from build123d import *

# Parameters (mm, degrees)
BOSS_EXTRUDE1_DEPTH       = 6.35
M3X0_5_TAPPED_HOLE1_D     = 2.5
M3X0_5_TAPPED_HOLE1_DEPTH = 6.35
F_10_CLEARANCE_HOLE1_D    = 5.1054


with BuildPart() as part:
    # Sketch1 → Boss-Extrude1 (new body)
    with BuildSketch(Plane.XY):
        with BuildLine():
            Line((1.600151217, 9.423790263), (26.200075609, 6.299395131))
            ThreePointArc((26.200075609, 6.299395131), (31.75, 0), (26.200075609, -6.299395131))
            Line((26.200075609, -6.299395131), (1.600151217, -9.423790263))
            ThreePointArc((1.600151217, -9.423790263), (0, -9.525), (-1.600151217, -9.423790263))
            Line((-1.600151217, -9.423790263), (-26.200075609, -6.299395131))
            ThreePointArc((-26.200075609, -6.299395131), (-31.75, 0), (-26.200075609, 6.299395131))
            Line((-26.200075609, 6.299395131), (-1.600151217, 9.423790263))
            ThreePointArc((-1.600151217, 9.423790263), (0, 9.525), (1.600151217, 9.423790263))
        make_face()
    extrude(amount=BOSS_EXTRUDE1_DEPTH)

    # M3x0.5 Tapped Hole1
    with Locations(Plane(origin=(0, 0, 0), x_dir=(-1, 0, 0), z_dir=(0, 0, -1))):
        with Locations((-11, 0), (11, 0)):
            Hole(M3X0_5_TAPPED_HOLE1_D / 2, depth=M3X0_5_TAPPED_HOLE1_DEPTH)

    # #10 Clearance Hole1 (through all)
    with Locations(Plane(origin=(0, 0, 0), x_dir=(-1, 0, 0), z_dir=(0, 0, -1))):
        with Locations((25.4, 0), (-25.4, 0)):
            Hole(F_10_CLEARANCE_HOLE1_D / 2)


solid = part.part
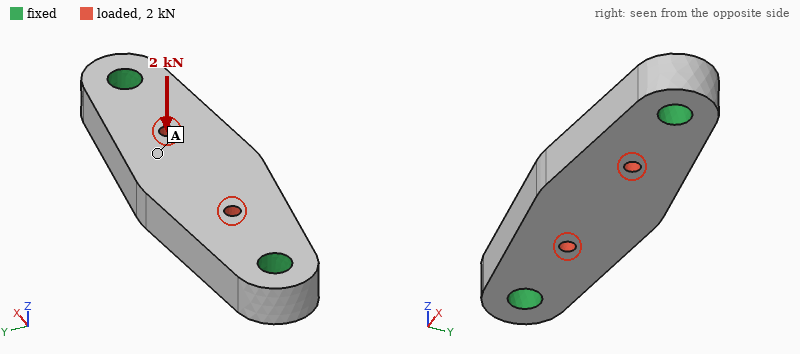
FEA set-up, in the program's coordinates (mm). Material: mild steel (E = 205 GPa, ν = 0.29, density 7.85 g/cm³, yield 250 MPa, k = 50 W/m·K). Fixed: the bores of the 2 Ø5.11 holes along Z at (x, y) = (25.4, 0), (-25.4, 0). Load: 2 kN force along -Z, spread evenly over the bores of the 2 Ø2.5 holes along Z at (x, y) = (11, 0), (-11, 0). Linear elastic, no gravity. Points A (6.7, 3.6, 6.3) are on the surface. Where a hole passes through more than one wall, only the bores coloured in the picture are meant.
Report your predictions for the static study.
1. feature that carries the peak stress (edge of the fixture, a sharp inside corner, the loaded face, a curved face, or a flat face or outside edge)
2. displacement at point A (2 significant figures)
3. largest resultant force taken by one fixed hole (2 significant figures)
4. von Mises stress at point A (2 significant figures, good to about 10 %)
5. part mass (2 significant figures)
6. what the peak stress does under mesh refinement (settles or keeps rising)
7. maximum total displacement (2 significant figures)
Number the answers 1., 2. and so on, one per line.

1. edge of the fixture
2. 11 µm
3. 1.0 kN
4. 35 MPa
5. 44 g
6. keeps rising
7. 12 µm
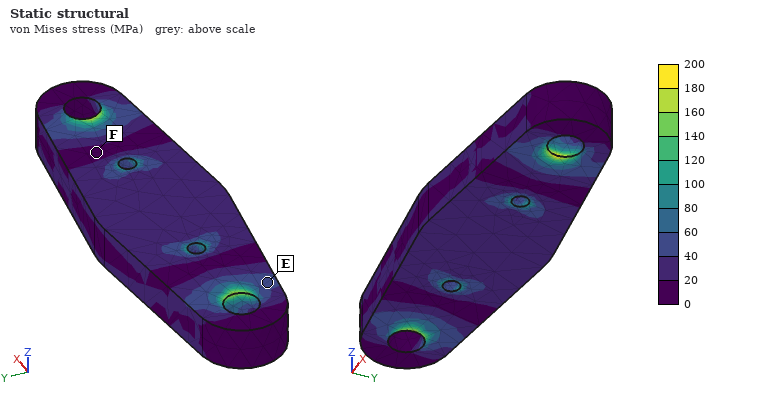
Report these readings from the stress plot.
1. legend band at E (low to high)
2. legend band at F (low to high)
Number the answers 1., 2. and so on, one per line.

1. 40 to 60 MPa
2. 0 to 20 MPa
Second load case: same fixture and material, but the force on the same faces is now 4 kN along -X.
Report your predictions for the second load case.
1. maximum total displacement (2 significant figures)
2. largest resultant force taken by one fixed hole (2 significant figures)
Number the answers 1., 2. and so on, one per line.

1. 2.2 µm
2. 2.0 kN
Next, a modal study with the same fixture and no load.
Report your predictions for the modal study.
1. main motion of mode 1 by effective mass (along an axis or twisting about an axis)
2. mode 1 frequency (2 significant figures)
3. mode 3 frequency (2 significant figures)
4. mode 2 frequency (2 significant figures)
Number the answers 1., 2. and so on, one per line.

1. along Z
2. 12 kHz
3. 19 kHz
4. 18 kHz
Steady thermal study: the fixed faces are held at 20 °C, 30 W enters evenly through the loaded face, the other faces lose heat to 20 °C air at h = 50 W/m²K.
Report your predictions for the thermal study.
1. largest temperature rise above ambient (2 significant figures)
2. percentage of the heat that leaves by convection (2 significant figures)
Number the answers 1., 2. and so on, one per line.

1. 48 K
2. 11 %
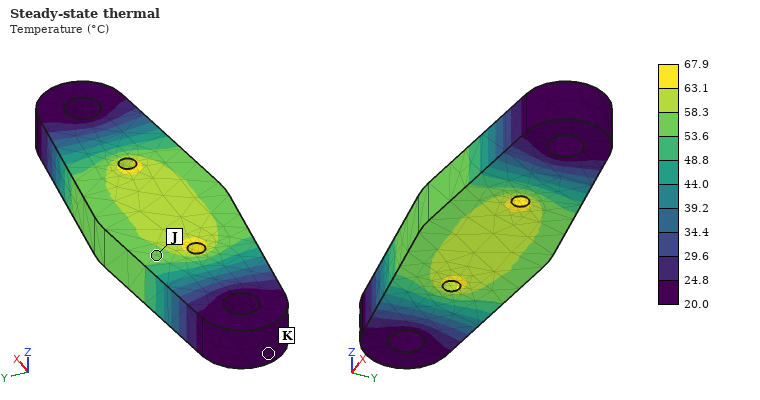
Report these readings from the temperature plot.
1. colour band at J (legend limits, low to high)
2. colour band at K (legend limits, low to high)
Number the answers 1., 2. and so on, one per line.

1. 53.6 to 58.3 °C
2. 20.0 to 24.8 °C
